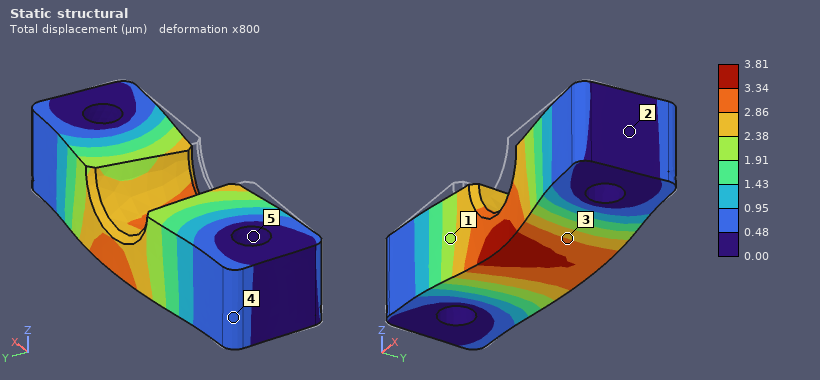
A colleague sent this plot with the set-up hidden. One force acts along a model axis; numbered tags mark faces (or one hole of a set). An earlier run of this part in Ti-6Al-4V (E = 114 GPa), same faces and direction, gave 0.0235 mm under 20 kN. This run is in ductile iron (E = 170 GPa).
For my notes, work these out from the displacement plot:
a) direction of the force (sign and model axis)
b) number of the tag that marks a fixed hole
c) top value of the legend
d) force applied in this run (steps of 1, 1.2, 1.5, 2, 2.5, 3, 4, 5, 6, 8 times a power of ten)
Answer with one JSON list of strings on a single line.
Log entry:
["+Y", "5", "3.81 µm", "5 kN"]
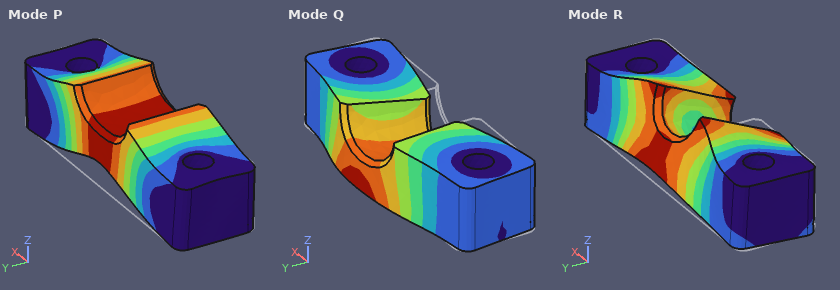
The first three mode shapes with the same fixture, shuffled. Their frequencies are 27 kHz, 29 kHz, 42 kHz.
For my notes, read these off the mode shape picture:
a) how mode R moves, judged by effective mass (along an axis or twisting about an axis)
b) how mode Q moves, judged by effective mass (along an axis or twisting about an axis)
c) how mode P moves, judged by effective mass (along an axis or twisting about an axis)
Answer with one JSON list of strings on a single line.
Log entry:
["twisting about X", "along Y", "along Z"]
